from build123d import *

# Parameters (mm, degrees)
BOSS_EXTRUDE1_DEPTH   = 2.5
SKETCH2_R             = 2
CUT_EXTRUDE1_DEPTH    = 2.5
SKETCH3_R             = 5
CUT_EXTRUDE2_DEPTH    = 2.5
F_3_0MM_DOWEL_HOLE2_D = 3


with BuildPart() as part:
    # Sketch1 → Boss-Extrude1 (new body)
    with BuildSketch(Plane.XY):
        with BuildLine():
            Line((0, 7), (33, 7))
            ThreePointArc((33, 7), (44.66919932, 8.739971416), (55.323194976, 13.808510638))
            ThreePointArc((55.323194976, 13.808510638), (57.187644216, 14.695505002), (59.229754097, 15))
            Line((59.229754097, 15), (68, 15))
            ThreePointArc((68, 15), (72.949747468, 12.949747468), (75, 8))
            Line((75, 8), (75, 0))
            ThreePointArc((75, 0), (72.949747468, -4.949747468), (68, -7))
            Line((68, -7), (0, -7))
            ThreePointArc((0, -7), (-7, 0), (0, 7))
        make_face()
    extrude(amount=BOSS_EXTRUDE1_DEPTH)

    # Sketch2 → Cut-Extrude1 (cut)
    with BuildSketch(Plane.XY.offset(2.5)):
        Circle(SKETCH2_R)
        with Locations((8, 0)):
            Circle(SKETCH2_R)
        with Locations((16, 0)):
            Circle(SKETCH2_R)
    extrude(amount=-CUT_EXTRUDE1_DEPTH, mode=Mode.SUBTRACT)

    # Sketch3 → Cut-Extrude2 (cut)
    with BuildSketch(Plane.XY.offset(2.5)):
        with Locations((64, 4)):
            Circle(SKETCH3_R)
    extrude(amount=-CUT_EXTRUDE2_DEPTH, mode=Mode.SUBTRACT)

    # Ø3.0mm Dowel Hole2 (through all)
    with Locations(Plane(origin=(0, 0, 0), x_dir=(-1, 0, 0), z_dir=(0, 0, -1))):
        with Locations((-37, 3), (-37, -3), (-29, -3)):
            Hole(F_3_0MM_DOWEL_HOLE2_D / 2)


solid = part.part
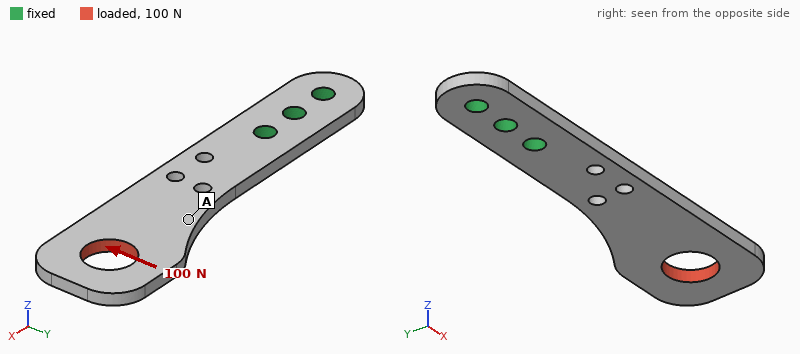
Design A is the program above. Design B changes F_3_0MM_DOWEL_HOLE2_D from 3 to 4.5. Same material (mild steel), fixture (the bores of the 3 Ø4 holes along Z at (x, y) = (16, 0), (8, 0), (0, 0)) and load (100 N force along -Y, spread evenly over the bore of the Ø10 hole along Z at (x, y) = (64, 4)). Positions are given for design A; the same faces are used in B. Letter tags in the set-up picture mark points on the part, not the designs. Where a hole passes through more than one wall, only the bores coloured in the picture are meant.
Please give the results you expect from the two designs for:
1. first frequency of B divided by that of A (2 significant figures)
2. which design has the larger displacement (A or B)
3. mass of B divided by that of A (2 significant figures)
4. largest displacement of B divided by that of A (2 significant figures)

0.94
B
0.98
1.1
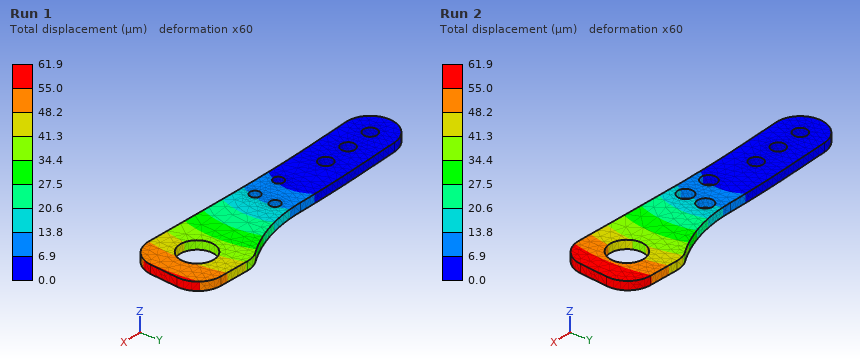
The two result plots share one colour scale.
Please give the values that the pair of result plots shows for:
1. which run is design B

Run 2
